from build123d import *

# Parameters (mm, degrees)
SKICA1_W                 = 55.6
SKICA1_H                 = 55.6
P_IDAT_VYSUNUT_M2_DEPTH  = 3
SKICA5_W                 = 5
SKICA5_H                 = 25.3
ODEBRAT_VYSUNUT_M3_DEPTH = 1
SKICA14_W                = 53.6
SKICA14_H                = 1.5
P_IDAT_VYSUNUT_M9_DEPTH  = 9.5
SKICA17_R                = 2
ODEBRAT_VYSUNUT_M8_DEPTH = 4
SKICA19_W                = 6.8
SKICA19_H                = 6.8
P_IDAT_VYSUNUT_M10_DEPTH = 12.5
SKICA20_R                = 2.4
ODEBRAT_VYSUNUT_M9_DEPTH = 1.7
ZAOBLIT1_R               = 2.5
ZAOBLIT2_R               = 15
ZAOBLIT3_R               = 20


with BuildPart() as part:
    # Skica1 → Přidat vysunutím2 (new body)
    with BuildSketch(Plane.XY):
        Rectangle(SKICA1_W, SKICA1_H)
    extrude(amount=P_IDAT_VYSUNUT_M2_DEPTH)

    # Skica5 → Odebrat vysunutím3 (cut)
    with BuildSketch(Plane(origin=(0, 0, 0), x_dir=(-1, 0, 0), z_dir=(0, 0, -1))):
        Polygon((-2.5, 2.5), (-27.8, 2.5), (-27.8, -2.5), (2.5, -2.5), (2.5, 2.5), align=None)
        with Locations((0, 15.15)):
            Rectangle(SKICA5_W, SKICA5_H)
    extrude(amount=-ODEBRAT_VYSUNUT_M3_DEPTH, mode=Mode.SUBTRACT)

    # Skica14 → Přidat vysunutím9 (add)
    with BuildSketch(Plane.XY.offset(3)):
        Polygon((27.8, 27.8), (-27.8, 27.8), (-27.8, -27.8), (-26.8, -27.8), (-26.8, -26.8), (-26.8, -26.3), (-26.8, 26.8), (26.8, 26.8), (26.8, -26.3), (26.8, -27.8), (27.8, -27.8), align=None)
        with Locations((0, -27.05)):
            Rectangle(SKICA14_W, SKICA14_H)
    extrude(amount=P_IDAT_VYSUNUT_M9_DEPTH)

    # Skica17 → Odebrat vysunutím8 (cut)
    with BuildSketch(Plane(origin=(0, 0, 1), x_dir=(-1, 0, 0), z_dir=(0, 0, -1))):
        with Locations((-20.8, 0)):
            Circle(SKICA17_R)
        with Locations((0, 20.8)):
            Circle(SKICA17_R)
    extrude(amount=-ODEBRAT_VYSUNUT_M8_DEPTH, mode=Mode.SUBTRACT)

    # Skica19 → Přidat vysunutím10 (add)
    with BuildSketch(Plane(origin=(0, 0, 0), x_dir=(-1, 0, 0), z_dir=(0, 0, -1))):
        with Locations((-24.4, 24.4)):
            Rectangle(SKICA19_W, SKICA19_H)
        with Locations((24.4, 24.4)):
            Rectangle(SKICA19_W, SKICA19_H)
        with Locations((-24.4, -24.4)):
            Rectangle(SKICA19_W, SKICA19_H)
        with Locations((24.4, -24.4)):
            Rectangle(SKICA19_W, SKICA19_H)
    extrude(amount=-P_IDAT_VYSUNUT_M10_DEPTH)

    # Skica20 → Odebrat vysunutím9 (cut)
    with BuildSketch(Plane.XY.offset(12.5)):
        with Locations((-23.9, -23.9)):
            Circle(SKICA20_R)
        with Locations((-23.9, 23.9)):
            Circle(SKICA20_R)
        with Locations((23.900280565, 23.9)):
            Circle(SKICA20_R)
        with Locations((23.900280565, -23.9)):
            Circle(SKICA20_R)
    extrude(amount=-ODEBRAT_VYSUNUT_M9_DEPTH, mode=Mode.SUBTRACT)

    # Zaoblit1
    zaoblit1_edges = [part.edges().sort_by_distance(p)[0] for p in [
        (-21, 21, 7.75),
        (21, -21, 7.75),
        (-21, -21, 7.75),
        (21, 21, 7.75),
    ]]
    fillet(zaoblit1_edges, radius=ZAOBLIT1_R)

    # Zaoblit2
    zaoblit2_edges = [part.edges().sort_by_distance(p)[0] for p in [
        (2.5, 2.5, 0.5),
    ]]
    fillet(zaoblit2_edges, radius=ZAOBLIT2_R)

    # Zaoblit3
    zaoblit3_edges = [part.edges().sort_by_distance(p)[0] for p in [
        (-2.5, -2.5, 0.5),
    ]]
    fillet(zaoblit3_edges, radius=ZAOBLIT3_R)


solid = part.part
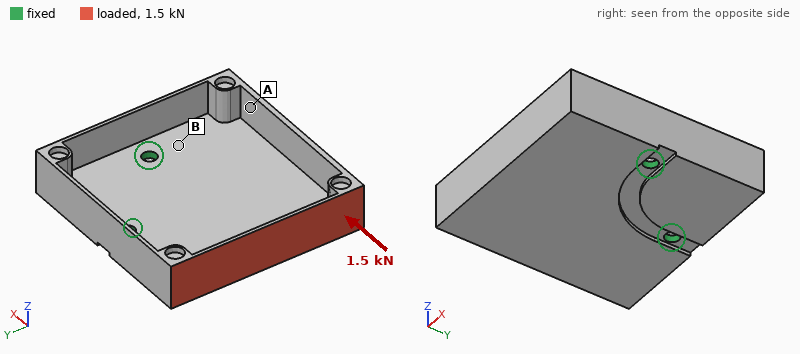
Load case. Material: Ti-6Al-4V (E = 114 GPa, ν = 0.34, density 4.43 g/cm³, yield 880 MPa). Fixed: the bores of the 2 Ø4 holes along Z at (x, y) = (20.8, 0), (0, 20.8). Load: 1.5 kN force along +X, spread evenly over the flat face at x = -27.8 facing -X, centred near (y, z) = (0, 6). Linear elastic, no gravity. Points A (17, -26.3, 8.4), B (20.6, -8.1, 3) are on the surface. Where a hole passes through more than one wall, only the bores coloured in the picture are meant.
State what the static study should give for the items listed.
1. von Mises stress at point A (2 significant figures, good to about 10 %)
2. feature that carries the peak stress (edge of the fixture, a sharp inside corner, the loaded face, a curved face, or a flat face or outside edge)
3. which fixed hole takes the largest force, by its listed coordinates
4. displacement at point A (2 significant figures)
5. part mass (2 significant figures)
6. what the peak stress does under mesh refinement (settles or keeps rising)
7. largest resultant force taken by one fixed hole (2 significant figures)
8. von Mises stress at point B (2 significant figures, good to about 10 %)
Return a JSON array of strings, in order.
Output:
["27 MPa", "edge of the fixture", "(20.8, 0)", "0.058 mm", "55 g", "keeps rising", "1.1 kN", "50 MPa"]
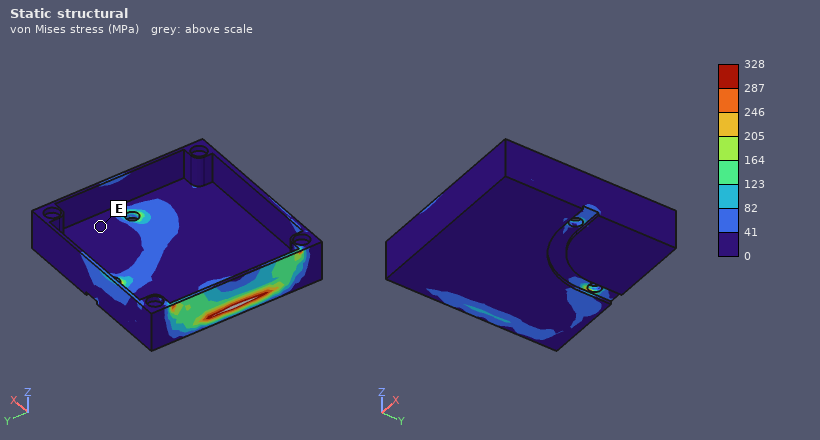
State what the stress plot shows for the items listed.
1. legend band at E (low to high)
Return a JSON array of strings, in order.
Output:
["0 to 41 MPa"]
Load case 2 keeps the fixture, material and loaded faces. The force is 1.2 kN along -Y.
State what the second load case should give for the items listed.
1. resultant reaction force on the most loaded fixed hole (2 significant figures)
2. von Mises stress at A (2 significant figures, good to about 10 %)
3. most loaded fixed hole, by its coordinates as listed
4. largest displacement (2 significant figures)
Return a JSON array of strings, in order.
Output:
["1.9 kN", "23 MPa", "(0, 20.8)", "0.39 mm"]
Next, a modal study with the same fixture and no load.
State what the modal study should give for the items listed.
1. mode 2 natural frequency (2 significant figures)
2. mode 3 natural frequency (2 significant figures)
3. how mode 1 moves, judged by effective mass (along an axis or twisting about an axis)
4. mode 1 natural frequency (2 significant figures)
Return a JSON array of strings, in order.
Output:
["2900 Hz", "3400 Hz", "along Z", "950 Hz"]
